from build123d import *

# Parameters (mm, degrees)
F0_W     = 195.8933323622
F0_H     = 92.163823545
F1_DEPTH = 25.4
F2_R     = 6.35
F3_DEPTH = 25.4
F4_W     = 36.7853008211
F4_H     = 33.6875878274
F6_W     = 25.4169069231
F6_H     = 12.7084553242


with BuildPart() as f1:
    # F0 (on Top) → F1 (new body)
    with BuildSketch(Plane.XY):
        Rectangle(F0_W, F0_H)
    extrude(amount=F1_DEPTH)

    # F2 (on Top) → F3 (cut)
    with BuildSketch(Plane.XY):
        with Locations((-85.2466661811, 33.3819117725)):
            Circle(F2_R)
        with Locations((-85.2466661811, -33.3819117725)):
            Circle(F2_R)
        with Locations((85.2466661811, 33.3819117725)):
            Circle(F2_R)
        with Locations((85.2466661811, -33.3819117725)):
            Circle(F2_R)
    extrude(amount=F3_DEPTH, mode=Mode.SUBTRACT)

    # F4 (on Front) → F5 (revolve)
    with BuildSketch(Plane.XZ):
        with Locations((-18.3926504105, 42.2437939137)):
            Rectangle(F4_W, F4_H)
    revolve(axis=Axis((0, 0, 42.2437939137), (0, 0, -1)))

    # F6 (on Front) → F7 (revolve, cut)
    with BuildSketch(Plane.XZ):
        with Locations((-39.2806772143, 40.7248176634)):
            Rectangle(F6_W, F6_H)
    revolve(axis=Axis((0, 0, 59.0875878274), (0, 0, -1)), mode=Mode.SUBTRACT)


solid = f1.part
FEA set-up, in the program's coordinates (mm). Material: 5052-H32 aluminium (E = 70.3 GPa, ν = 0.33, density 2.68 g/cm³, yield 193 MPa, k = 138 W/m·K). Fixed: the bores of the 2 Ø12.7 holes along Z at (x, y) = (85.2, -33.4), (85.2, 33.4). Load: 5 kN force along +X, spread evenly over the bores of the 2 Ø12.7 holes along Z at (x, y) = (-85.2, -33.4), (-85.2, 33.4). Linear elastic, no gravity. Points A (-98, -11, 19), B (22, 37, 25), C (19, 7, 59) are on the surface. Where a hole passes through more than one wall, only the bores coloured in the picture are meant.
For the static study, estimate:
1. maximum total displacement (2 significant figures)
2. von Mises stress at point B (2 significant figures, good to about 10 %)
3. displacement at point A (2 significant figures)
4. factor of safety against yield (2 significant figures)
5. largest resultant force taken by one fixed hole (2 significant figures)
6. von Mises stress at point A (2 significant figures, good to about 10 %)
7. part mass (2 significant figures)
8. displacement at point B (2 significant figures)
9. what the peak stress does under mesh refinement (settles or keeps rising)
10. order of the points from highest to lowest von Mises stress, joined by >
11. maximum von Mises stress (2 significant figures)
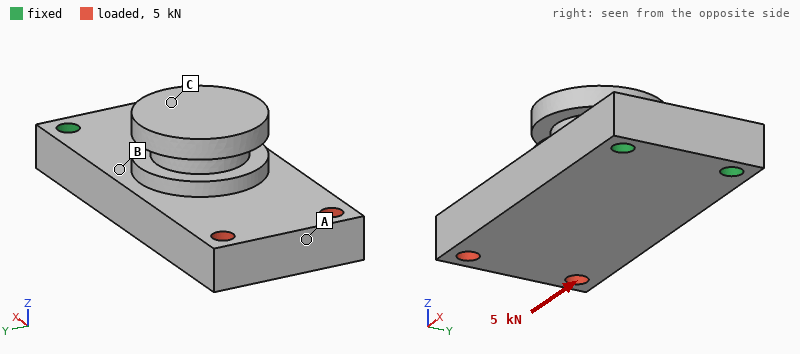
8.7 µm
1.7 MPa
6.3 µm
20
2.6 kN
2.8 MPa
1.5 kg
2.1 µm
settles
A > B > C
9.5 MPa
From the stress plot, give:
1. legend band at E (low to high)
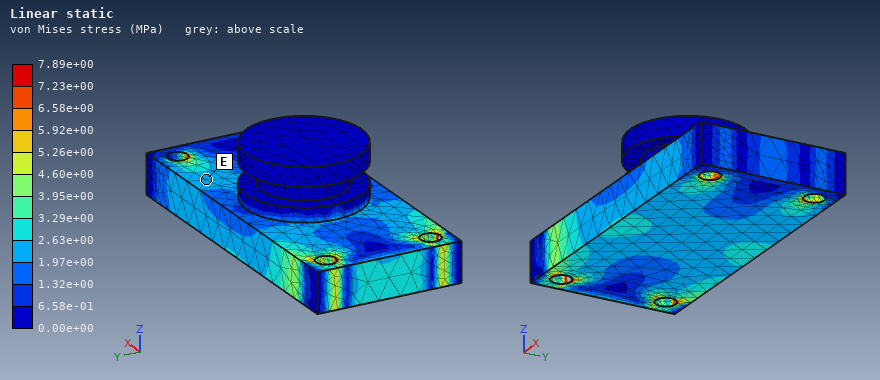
1.97e+00 to 2.63e+00 MPa
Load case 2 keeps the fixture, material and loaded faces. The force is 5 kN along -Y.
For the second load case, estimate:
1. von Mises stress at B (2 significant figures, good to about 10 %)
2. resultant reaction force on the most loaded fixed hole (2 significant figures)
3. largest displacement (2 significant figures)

13 MPa
12 kN
97 µm
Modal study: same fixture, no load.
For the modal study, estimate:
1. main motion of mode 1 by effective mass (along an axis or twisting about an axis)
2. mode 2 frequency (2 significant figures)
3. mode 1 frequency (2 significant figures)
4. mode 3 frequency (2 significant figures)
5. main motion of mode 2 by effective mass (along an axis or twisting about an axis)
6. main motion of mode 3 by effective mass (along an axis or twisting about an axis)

along Z
1900 Hz
600 Hz
2400 Hz
along Y
twisting about X
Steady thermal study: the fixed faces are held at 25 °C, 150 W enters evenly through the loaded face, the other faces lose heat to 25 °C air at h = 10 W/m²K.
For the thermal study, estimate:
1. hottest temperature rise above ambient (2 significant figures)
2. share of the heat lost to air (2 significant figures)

75 K
14 %
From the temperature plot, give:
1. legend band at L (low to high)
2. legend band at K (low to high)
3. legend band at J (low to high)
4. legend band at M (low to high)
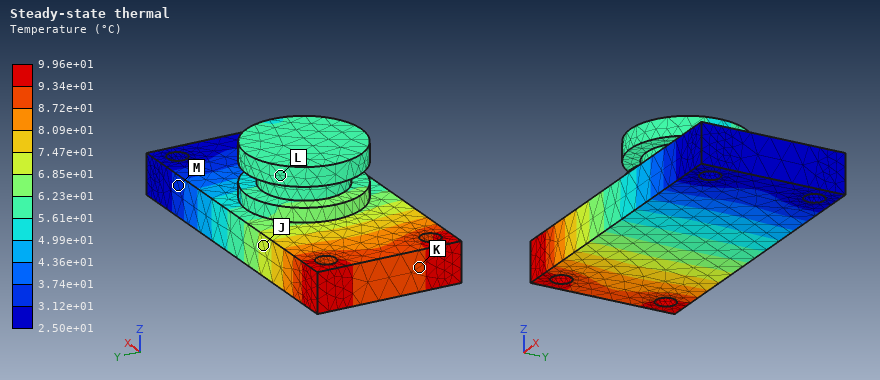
5.61e+01 to 6.23e+01 °C
8.72e+01 to 9.34e+01 °C
6.85e+01 to 7.47e+01 °C
3.12e+01 to 3.74e+01 °C
